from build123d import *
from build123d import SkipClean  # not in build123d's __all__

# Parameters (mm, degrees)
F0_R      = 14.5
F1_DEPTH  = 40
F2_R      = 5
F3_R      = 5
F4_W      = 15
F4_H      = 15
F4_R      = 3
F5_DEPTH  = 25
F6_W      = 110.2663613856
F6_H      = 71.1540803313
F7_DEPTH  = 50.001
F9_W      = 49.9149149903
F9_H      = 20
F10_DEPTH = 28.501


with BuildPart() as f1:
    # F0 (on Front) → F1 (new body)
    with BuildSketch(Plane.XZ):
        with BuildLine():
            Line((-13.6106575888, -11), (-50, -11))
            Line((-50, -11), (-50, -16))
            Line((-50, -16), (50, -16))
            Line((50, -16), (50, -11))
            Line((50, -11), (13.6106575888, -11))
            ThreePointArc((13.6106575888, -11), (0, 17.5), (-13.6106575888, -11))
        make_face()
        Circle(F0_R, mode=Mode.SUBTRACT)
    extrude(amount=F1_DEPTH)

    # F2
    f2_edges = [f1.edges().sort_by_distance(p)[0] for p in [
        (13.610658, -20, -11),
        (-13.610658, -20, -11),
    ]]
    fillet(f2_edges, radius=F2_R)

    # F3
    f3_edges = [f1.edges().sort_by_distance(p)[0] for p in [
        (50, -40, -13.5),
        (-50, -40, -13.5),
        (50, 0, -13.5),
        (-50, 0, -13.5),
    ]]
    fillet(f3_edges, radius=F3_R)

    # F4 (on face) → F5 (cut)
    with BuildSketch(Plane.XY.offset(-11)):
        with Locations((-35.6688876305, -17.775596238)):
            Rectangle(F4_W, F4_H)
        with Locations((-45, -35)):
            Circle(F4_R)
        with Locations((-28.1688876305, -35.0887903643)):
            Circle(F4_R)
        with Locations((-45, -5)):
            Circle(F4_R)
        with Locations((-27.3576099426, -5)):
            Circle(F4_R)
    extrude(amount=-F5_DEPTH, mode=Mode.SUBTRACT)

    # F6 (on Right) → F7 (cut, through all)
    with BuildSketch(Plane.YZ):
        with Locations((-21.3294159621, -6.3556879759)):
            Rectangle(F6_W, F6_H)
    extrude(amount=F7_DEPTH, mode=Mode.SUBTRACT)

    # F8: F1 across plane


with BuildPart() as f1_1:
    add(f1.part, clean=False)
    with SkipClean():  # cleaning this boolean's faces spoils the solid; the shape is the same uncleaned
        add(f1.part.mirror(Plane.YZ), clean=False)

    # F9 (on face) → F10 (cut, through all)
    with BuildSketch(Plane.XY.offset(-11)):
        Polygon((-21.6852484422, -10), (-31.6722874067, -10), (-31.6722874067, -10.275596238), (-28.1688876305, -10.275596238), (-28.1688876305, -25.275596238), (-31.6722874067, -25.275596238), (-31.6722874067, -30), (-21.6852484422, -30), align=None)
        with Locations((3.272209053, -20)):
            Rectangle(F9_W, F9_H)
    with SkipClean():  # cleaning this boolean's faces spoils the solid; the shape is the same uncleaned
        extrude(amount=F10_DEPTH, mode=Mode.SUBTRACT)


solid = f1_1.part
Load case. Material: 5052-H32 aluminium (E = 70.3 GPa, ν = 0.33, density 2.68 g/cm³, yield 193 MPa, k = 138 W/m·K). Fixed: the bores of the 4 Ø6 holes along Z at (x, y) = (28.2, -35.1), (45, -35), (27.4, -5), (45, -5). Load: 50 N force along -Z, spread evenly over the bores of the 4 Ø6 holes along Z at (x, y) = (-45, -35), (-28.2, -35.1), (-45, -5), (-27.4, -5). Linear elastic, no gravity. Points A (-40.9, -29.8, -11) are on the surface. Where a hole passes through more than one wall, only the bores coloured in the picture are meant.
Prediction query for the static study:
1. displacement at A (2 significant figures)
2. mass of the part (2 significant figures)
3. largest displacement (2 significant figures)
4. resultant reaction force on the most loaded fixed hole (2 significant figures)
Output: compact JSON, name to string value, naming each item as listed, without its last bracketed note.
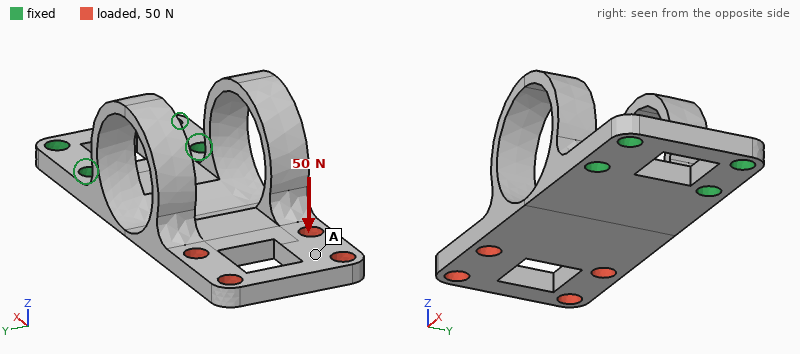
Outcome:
{"displacement at A": "0.21 mm", "mass of the part": "53 g", "largest displacement": "0.25 mm", "resultant reaction force on the most loaded fixed hole": "35 N"}
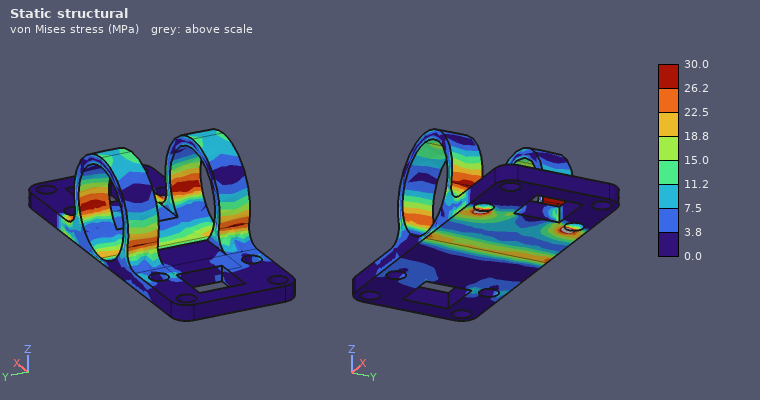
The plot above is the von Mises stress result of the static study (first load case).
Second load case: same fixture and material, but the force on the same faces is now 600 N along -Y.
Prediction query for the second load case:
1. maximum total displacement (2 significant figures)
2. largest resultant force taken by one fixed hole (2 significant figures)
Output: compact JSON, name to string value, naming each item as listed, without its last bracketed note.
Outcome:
{"maximum total displacement": "88 µm", "largest resultant force taken by one fixed hole": "1.2 kN"}
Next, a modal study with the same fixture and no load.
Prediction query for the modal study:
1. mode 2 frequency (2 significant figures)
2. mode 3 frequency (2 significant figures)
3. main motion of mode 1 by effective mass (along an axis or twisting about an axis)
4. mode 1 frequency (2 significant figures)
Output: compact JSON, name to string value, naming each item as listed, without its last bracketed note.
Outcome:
{"mode 2 frequency": "2000 Hz", "mode 3 frequency": "3500 Hz", "main motion of mode 1 by effective mass": "along Z", "mode 1 frequency": "660 Hz"}
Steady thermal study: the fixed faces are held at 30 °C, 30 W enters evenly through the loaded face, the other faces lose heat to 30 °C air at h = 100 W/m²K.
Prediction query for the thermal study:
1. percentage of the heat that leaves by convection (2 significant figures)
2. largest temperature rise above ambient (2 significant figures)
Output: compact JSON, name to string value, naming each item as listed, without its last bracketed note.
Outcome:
{"percentage of the heat that leaves by convection": "67 %", "largest temperature rise above ambient": "54 K"}
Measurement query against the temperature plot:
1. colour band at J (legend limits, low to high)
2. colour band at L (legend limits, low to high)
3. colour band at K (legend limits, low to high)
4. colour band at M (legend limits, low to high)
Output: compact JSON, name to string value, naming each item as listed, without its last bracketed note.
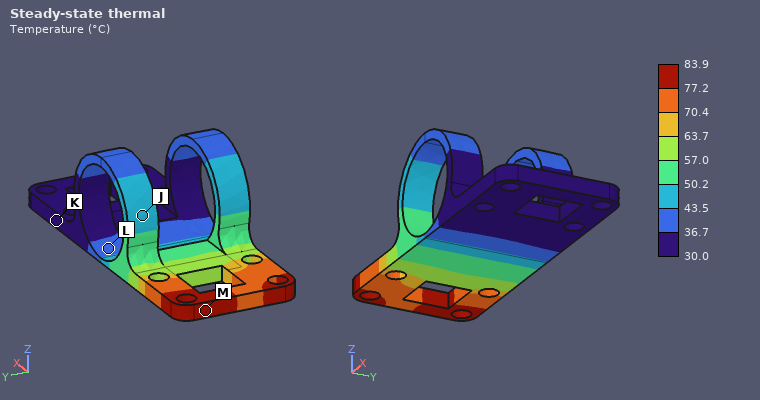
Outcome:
{"colour band at J": "43.5 to 50.2 °C", "colour band at L": "36.7 to 43.5 °C", "colour band at K": "30.0 to 36.7 °C", "colour band at M": "77.2 to 83.9 °C"}
